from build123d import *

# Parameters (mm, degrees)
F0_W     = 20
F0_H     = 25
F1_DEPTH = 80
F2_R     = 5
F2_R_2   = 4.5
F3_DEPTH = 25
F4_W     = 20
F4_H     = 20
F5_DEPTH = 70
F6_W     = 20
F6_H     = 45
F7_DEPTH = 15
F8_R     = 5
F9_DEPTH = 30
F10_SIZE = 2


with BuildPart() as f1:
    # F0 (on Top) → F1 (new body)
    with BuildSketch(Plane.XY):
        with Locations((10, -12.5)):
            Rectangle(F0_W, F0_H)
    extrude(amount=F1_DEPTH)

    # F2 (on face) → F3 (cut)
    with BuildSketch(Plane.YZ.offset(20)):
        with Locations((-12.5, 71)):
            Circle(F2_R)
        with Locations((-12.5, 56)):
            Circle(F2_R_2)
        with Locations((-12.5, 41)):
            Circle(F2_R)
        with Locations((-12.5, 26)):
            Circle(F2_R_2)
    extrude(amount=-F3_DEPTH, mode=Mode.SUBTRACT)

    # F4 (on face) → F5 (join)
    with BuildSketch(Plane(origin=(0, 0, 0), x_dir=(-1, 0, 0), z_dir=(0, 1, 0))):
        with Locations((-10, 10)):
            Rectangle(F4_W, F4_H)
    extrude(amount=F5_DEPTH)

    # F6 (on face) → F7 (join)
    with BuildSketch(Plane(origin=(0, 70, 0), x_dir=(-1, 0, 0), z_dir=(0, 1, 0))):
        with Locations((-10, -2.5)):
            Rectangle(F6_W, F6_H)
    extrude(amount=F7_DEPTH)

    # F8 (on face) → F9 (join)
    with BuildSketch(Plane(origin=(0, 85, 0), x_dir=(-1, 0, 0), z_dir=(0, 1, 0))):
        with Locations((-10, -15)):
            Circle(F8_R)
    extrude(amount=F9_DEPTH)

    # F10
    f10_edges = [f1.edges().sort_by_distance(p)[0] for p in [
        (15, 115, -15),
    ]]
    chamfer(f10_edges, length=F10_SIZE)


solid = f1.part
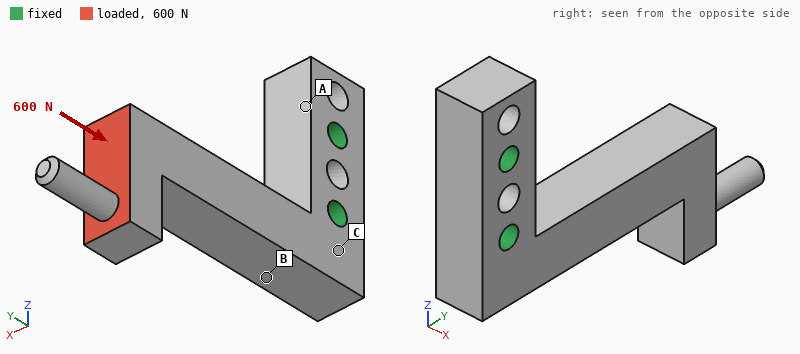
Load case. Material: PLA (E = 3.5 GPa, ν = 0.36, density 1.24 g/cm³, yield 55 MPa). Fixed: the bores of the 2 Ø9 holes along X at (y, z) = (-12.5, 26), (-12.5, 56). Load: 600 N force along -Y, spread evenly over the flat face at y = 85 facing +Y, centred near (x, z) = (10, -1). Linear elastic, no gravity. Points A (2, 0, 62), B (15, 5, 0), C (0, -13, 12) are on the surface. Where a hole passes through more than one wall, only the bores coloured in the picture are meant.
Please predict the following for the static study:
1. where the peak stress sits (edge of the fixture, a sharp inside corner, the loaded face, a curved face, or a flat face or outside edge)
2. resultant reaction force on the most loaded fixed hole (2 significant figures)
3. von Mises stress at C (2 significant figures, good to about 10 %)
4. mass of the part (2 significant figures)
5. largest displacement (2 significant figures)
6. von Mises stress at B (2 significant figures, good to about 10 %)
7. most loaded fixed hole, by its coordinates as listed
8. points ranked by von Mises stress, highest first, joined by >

edge of the fixture
760 N
4.4 MPa
97 g
1.6 mm
6.7 MPa
(-12.5, 26)
B > C > A
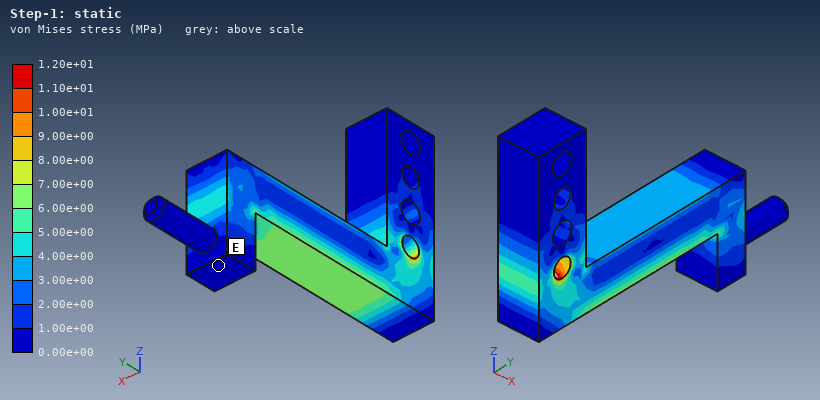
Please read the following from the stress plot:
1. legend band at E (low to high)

0.00e+00 to 1.00e+00 MPa
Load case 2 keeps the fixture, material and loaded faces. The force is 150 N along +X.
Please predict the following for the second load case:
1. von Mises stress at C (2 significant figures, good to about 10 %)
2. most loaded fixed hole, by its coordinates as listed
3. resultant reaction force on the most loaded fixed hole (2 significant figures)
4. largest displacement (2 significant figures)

5.4 MPa
(-12.5, 26)
160 N
1.8 mm
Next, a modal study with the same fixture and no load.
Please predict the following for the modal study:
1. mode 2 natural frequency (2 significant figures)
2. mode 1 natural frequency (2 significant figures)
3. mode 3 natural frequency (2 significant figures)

350 Hz
350 Hz
1200 Hz
